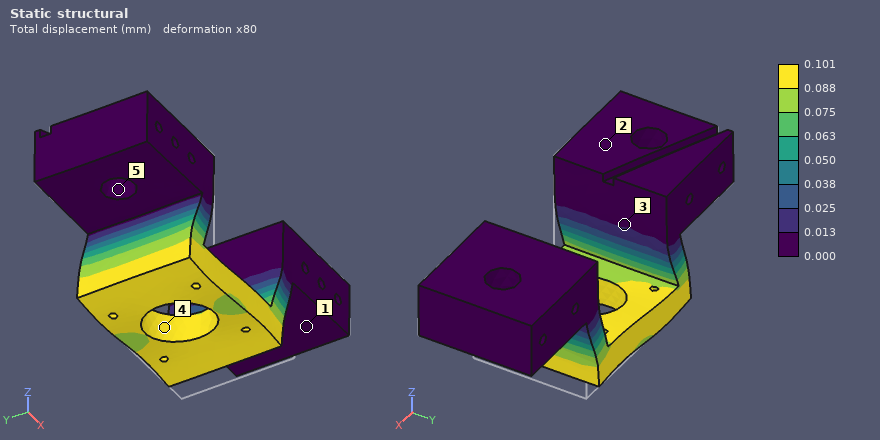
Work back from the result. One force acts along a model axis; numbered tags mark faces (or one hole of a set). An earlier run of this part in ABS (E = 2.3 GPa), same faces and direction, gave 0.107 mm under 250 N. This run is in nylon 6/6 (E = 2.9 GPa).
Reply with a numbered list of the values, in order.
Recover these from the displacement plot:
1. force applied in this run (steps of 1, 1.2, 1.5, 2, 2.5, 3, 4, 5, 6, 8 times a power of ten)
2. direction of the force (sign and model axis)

1. 300 N
2. -X
